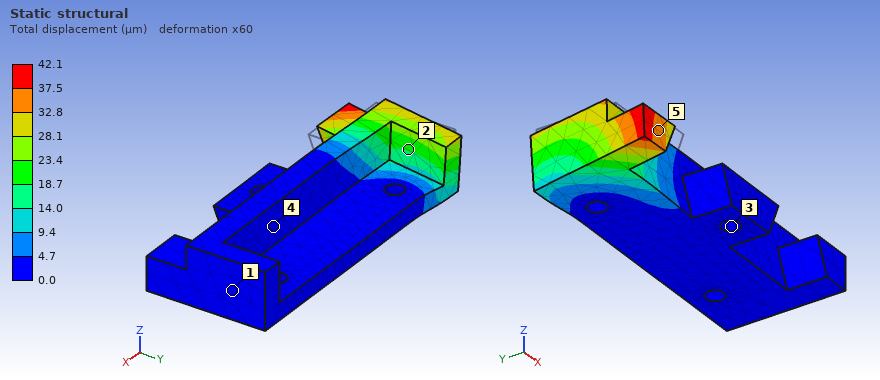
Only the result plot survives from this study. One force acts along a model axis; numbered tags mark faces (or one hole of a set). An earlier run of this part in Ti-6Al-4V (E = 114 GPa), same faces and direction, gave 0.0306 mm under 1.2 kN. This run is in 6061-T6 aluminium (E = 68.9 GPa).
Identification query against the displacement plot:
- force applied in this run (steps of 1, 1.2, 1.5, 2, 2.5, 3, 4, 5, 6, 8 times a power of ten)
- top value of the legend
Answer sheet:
1 kN
42.1 µm
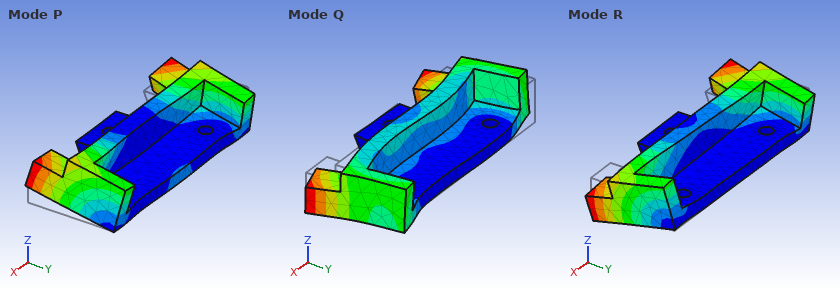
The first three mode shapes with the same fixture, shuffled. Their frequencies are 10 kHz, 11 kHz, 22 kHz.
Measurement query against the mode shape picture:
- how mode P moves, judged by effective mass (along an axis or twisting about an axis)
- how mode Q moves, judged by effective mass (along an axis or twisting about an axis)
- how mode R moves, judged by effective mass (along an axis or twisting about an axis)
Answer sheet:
along Z
along X
twisting about Y
